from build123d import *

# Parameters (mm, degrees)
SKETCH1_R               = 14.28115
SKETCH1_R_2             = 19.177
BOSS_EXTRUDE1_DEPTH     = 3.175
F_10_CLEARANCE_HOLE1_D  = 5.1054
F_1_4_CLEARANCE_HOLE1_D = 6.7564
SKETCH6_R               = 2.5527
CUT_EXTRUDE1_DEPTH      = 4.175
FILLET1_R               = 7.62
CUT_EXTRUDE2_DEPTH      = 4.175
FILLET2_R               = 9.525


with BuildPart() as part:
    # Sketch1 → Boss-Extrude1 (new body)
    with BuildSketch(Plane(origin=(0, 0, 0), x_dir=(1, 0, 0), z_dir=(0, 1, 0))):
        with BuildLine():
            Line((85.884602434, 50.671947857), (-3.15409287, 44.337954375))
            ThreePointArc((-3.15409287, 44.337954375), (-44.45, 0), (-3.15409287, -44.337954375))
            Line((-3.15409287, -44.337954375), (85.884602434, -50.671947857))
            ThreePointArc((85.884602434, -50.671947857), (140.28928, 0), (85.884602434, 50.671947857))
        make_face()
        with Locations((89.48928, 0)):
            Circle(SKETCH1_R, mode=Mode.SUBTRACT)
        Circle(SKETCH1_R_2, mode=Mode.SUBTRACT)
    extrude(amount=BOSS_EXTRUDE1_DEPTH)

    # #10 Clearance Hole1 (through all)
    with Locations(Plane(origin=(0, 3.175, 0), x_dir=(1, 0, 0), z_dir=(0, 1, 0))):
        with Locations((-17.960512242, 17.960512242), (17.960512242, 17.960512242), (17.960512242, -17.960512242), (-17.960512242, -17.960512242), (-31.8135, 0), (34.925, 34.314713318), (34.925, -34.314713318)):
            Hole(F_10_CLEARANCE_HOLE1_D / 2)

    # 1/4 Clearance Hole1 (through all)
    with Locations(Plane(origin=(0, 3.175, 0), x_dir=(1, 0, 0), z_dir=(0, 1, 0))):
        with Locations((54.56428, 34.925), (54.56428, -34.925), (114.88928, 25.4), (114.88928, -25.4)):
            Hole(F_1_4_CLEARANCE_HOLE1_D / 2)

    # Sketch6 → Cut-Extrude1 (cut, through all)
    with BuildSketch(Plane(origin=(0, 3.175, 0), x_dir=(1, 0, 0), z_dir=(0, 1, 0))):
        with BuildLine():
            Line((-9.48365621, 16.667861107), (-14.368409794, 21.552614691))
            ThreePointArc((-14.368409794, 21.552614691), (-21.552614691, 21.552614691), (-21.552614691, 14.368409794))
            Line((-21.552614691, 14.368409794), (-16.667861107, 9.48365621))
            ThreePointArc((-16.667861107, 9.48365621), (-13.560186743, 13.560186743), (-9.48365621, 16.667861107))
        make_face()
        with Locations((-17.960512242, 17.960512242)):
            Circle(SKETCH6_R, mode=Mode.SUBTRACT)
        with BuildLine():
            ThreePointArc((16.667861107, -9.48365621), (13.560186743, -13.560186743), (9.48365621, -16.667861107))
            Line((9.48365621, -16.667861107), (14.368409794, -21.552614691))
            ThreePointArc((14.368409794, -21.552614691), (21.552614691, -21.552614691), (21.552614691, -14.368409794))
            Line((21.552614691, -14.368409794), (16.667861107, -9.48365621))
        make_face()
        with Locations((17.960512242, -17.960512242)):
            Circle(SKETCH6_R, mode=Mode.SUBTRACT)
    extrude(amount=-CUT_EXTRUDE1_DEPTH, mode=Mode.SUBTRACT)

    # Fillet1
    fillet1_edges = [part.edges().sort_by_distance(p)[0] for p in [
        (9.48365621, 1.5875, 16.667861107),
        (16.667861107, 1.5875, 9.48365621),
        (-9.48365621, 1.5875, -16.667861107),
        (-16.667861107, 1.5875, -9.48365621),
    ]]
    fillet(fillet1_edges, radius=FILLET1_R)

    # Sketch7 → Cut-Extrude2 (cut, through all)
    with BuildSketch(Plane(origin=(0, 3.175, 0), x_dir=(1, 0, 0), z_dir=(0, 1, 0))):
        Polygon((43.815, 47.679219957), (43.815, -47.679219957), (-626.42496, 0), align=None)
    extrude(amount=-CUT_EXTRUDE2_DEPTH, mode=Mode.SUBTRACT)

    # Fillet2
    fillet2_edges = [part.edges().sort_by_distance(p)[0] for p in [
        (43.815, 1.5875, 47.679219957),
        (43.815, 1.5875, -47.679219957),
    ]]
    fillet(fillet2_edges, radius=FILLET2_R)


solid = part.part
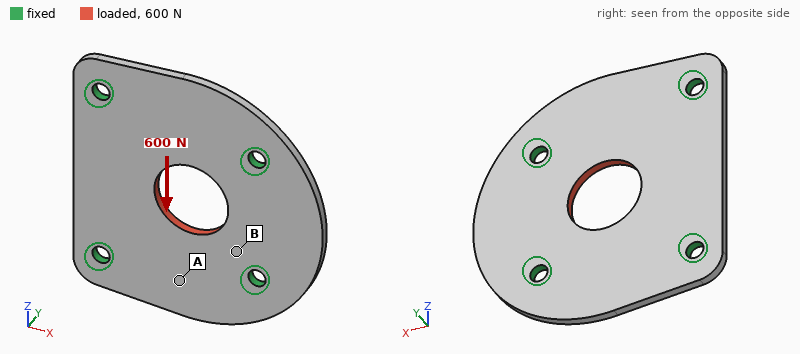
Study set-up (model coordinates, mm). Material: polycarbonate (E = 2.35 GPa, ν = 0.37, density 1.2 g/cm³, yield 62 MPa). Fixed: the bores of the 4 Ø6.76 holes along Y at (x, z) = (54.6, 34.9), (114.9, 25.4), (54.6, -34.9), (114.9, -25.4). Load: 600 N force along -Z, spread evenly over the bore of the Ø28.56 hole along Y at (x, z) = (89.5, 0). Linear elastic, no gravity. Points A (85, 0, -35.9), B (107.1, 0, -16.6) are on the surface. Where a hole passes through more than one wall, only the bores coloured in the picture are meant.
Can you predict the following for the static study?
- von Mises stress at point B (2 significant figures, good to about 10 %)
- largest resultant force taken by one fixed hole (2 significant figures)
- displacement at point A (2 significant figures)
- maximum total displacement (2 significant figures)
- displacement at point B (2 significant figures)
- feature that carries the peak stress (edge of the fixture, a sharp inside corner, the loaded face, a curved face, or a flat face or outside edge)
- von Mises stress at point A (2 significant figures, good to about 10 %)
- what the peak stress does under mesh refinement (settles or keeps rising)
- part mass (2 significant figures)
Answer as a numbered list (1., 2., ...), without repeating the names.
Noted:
1. 2.4 MPa
2. 170 N
3. 29 µm
4. 41 µm
5. 15 µm
6. edge of the fixture
7. 0.79 MPa
8. keeps rising
9. 29 g
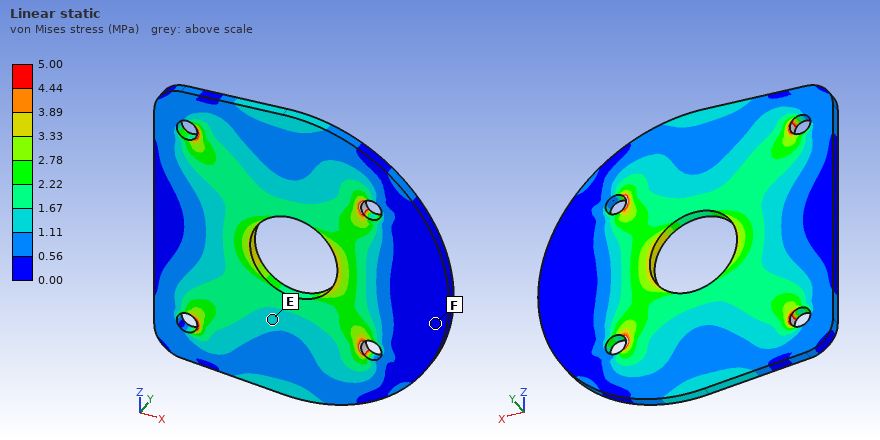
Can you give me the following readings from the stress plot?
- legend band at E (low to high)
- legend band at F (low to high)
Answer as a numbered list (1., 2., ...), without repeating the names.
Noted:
1. 1.11 to 1.67 MPa
2. 0.00 to 0.56 MPa
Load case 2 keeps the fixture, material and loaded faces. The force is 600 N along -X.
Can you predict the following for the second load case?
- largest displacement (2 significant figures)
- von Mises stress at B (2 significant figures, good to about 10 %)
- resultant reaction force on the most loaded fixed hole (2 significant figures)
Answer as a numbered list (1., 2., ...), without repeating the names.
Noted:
1. 48 µm
2. 2.6 MPa
3. 190 N
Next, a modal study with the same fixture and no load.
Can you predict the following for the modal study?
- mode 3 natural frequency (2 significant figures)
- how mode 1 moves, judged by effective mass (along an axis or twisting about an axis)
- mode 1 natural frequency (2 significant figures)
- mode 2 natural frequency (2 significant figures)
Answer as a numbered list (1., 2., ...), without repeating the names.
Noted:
1. 1100 Hz
2. along Y
3. 970 Hz
4. 1100 Hz
